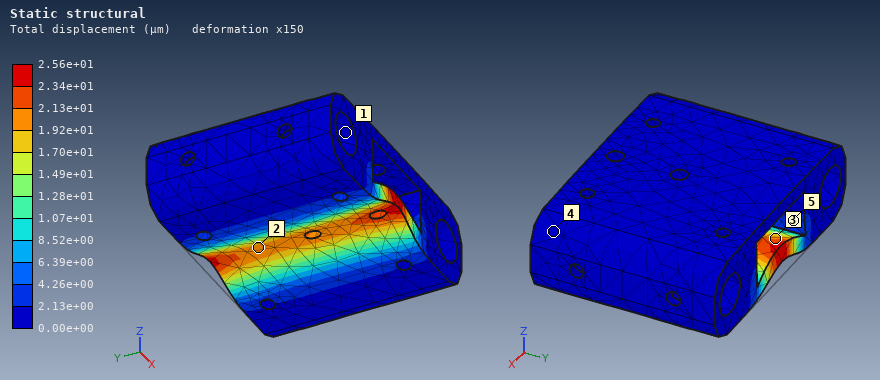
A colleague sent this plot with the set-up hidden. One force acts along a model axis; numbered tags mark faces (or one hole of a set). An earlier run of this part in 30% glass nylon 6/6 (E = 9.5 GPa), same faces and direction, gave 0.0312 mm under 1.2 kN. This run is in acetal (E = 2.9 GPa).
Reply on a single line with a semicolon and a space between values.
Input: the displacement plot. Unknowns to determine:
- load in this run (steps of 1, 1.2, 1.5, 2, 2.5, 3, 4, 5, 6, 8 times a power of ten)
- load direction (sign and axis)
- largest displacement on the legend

300 N; +Z; 2.56e+01 µm
